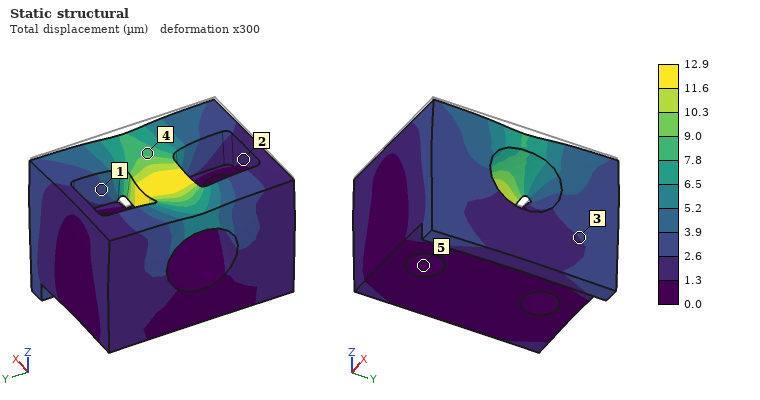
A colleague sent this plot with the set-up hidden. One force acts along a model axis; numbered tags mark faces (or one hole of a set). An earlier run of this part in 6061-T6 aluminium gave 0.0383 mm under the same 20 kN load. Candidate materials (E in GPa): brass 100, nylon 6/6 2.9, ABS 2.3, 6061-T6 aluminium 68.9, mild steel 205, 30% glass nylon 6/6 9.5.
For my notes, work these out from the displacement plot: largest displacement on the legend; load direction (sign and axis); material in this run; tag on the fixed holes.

12.9 µm
-Z
mild steel
5
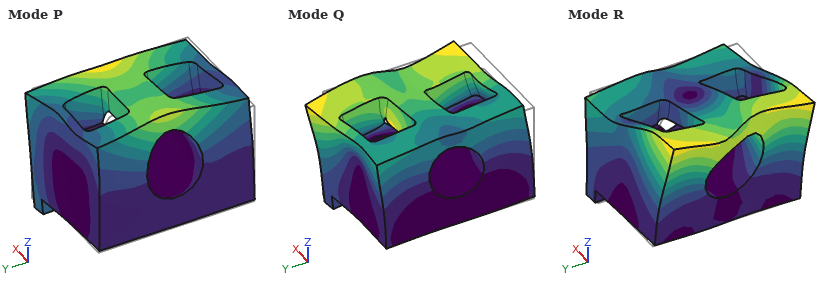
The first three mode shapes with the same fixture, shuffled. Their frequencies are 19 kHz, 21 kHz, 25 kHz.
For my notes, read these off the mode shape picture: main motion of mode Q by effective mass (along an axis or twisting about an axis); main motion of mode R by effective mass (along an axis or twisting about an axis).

along Y
twisting about Z
